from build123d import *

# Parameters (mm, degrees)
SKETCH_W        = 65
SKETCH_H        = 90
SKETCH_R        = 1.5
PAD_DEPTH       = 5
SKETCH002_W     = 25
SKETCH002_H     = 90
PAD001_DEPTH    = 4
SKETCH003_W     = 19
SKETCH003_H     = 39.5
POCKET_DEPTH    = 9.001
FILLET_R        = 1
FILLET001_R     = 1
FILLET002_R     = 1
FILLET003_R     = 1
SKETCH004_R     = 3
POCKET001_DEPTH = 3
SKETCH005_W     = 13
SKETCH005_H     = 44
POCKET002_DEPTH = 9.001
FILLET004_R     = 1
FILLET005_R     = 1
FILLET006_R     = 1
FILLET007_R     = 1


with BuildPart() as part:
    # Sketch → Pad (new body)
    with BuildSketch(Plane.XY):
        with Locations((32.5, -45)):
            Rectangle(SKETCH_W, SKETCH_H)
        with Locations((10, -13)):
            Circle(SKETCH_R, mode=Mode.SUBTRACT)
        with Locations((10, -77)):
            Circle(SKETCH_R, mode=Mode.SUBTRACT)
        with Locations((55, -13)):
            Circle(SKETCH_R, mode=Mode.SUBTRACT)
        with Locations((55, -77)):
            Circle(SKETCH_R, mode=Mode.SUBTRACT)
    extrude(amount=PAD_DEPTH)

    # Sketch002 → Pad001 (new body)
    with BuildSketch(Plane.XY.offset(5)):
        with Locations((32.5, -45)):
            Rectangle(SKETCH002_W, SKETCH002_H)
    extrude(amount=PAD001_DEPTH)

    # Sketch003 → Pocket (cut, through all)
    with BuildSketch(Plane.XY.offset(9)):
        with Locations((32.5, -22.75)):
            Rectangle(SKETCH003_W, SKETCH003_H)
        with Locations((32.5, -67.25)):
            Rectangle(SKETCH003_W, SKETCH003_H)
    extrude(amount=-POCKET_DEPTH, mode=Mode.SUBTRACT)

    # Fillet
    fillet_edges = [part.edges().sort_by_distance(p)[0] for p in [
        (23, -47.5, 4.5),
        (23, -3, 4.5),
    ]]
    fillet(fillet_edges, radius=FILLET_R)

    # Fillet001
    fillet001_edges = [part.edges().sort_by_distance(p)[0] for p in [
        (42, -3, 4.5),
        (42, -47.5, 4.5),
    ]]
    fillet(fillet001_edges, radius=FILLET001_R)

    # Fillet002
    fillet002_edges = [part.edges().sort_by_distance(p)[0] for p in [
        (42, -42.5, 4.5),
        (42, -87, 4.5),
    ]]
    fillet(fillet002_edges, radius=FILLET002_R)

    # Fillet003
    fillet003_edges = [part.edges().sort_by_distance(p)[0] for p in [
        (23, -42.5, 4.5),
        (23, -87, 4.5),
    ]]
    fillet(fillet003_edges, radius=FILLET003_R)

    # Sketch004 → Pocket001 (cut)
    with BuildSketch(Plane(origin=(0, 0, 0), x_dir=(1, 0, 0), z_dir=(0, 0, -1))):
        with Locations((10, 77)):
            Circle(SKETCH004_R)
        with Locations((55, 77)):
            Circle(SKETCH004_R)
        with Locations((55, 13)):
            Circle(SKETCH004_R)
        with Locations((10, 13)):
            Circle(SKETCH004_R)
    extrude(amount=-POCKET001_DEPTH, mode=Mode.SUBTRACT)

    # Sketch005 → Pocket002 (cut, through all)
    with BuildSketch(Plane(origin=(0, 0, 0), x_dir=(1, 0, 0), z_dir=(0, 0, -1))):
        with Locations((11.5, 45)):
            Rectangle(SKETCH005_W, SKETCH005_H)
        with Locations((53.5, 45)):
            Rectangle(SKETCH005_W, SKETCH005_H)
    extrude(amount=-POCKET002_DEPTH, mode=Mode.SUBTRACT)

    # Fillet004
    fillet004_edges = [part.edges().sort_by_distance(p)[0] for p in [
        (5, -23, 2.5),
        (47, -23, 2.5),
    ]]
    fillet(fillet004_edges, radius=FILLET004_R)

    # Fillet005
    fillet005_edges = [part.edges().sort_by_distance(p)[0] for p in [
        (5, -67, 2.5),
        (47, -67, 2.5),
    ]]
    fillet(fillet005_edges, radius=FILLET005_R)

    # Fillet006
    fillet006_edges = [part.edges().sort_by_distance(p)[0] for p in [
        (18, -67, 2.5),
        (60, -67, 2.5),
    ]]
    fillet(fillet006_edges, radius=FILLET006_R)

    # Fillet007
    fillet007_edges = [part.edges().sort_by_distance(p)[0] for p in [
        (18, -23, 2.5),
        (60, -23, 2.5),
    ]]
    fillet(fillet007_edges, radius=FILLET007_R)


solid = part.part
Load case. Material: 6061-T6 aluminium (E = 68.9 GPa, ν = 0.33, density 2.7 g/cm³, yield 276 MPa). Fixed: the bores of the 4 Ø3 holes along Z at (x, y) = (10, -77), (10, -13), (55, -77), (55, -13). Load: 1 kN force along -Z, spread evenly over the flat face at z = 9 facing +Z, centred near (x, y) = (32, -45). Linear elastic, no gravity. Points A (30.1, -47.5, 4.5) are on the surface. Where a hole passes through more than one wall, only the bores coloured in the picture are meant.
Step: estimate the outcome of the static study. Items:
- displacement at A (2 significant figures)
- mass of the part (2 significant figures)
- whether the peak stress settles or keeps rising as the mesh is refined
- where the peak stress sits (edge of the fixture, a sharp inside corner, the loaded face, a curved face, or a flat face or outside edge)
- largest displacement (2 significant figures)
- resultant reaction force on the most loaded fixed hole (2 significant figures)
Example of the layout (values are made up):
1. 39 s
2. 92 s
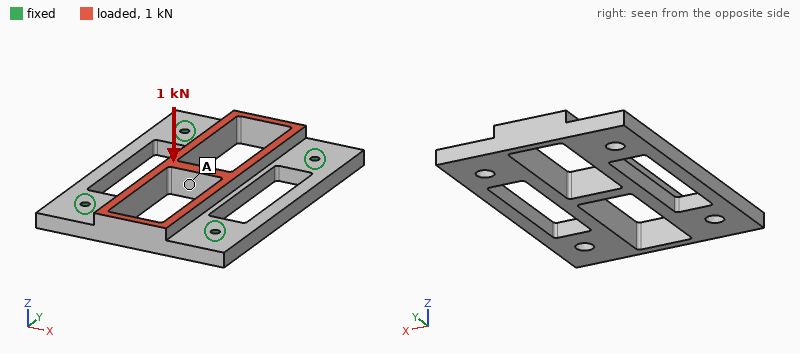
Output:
1. 59 µm
2. 50 g
3. keeps rising
4. edge of the fixture
5. 59 µm
6. 250 N
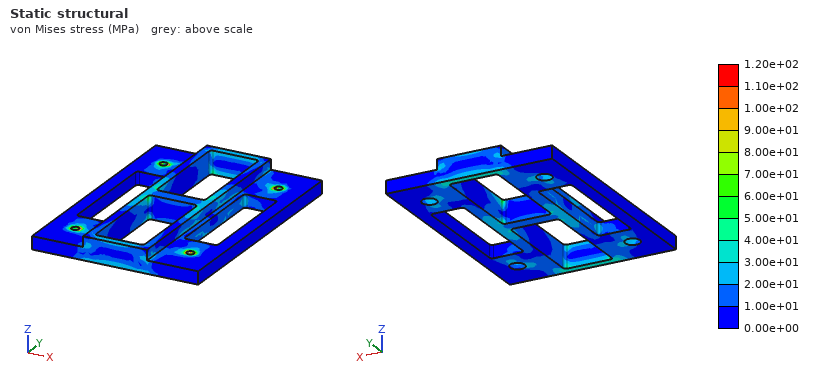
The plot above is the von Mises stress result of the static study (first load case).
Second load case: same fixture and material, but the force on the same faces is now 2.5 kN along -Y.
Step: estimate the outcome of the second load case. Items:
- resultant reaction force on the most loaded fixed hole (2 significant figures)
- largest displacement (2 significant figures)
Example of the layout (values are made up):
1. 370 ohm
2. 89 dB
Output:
1. 720 N
2. 35 µm
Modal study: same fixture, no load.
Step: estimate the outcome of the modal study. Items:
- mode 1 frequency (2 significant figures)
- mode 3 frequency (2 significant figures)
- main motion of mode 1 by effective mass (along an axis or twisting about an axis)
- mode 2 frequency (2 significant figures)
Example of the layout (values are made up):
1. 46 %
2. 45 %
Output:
1. 4500 Hz
2. 5600 Hz
3. along Z
4. 5300 Hz
